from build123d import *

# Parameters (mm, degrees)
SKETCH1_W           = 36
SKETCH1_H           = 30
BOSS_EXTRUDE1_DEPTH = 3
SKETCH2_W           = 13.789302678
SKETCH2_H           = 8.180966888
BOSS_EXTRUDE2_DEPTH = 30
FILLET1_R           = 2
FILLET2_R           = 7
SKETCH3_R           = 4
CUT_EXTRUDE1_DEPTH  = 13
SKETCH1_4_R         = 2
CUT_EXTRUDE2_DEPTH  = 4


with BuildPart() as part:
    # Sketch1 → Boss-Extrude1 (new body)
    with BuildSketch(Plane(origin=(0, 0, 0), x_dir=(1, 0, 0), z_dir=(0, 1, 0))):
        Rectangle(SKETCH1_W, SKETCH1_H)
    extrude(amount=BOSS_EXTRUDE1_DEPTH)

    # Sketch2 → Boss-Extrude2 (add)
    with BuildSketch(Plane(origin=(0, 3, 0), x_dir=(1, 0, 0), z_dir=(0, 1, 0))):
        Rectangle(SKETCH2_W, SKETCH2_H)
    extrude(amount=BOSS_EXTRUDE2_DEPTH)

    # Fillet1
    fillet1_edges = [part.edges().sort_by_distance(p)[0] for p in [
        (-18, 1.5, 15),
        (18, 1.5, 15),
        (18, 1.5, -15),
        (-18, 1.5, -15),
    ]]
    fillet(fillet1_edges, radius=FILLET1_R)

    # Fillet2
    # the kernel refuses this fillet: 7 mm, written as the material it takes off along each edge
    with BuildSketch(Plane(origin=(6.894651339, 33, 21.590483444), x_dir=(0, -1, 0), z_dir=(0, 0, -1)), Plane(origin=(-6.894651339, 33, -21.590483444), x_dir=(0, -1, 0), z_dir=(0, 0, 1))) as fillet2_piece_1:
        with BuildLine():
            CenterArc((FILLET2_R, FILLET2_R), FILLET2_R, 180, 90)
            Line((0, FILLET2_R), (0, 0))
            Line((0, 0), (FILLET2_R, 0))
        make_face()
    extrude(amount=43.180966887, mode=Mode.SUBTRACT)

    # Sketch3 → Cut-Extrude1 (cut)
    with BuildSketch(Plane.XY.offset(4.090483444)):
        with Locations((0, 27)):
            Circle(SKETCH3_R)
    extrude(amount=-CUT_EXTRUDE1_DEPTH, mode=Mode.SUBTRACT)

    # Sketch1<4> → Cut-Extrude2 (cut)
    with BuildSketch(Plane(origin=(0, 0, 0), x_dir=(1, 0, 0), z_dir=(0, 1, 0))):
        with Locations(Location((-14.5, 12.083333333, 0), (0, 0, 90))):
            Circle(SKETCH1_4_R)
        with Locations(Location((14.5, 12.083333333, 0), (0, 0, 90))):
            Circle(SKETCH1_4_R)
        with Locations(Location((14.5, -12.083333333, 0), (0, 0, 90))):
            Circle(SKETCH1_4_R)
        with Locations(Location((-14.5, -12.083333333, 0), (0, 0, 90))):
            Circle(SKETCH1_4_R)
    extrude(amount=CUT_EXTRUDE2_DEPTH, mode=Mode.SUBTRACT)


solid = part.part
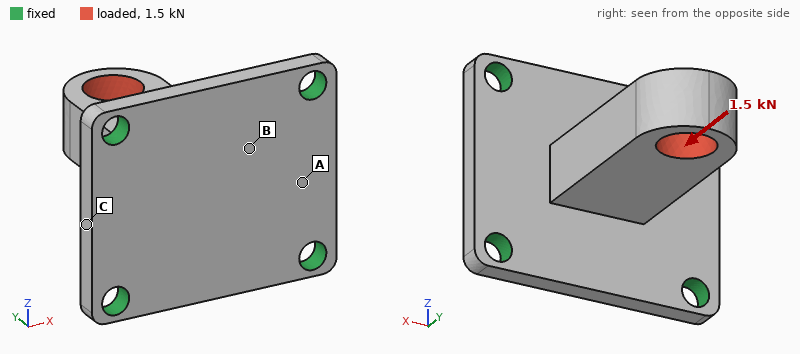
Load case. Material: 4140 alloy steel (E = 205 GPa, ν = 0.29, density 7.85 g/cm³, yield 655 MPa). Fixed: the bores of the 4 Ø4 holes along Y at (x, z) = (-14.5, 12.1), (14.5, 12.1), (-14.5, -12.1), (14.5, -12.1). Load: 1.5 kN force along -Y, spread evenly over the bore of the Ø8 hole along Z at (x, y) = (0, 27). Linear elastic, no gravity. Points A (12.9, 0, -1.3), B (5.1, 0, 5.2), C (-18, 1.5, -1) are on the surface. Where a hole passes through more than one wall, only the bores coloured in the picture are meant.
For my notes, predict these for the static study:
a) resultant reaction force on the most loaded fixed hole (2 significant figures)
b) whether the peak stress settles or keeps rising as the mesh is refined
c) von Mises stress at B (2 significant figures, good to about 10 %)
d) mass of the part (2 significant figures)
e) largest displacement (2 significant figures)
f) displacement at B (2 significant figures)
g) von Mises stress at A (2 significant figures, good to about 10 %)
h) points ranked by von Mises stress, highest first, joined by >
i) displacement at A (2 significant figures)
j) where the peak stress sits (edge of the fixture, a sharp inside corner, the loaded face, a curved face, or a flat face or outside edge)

390 N
keeps rising
60 MPa
46 g
16 µm
11 µm
42 MPa
B > A > C
6.1 µm
edge of the fixture
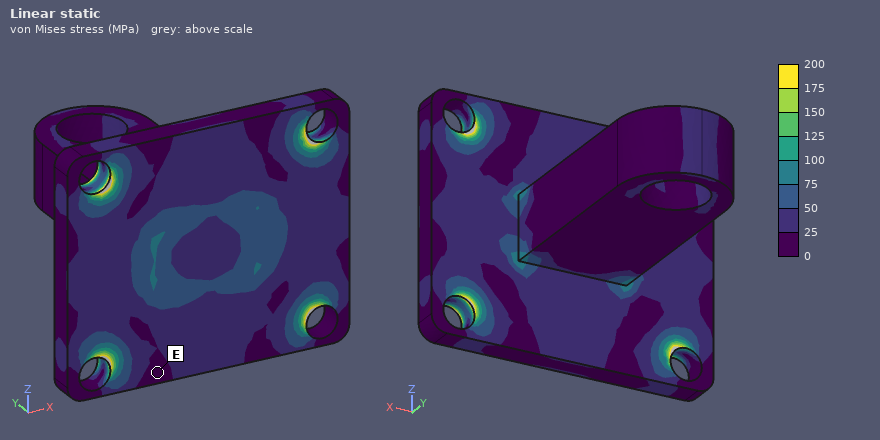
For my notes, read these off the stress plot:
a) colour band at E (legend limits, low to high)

0 to 25 MPa
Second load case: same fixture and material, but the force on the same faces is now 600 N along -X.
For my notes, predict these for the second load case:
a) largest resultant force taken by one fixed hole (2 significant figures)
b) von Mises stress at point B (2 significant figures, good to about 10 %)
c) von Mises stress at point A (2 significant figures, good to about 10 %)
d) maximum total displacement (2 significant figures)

370 N
70 MPa
43 MPa
51 µm
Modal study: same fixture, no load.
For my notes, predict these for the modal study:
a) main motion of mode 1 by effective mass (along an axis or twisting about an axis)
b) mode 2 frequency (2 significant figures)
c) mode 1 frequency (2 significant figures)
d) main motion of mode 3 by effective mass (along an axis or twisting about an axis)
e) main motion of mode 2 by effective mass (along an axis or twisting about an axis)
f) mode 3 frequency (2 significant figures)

along Z
6400 Hz
5000 Hz
along Y
along X
9800 Hz
